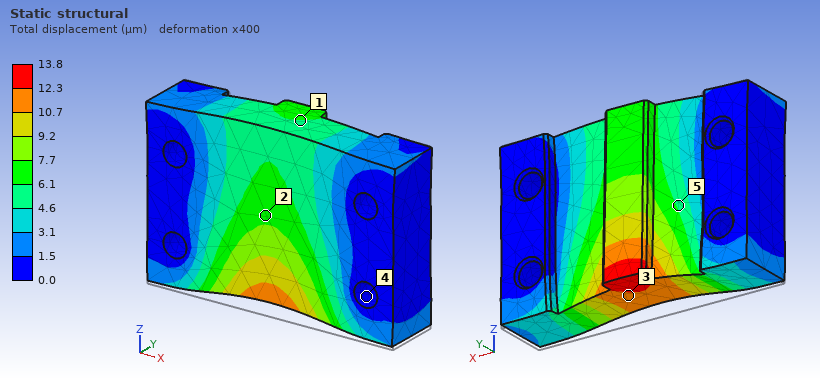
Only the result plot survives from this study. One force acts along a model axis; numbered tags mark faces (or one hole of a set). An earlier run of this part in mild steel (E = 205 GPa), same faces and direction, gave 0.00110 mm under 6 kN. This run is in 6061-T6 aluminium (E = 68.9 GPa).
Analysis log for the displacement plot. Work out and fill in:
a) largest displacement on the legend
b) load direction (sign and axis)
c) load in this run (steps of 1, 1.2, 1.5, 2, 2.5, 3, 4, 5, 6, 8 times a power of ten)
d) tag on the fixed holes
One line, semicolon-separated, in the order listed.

13.8 µm; +Z; 25 kN; 4
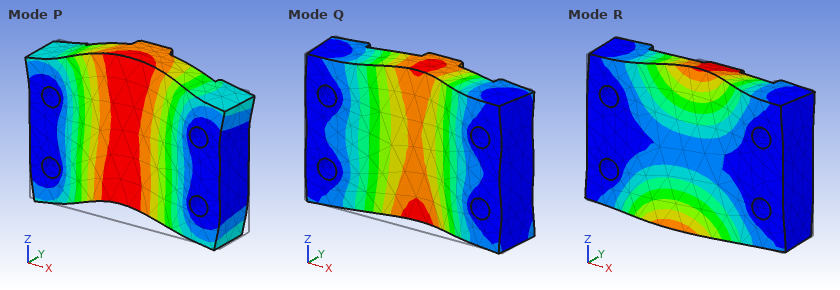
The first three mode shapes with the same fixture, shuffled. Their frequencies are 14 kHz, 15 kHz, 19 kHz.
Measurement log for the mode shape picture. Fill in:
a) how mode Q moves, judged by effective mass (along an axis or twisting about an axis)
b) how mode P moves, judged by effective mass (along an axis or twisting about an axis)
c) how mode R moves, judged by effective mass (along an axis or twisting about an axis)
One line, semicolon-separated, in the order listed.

along Y; along Z; twisting about X
